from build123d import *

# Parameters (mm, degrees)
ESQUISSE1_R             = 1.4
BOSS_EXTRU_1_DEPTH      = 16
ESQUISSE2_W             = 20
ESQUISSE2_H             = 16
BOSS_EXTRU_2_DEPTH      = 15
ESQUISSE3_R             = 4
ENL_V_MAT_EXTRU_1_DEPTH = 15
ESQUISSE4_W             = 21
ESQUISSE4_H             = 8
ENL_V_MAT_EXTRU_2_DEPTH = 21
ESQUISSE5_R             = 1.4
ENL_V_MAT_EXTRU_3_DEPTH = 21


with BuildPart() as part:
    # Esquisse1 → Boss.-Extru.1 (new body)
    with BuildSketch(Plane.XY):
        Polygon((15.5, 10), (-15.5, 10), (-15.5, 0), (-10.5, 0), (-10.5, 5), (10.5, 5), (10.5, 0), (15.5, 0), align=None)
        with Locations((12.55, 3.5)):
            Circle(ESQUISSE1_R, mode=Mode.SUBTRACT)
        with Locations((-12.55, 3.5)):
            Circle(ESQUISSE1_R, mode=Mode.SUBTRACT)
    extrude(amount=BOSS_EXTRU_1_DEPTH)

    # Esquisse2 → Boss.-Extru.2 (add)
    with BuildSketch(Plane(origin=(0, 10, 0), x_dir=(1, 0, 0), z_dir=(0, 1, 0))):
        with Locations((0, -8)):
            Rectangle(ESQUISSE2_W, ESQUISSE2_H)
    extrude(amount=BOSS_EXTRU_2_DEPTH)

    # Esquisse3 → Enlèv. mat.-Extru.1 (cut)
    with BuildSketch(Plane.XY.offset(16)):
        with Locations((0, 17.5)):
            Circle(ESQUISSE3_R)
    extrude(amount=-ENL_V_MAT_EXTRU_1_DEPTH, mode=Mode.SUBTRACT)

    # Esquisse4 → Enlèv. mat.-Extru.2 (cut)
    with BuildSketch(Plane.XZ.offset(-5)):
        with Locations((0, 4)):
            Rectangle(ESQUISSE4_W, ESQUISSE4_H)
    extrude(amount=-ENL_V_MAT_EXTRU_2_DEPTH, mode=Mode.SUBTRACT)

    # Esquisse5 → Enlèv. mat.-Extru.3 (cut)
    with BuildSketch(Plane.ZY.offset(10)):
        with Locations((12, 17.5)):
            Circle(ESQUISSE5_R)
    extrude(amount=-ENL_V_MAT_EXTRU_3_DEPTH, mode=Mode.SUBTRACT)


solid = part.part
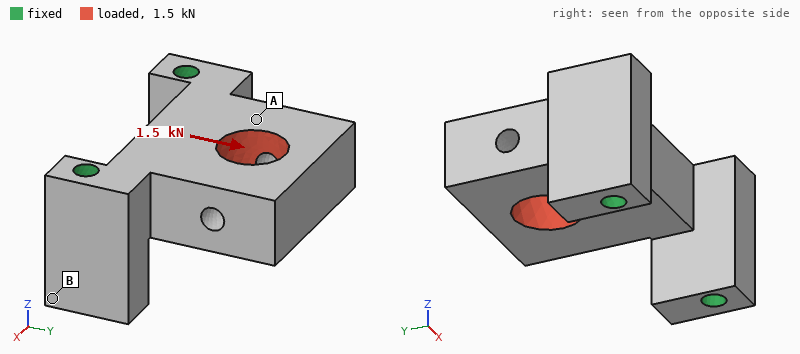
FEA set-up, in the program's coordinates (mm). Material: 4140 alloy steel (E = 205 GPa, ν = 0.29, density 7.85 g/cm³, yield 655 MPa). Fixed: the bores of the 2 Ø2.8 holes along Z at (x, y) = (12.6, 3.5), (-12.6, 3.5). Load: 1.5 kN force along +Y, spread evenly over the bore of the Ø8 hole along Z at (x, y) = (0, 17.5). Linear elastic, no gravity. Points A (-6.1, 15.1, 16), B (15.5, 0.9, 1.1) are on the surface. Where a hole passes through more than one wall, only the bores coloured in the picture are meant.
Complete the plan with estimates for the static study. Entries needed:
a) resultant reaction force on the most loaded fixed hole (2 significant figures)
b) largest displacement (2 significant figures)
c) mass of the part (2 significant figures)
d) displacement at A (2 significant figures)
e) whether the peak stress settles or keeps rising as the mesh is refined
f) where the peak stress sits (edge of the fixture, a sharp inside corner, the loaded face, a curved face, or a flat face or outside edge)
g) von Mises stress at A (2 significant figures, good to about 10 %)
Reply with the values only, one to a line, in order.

880 N
2.8 µm
33 g
1.9 µm
keeps rising
edge of the fixture
17 MPa
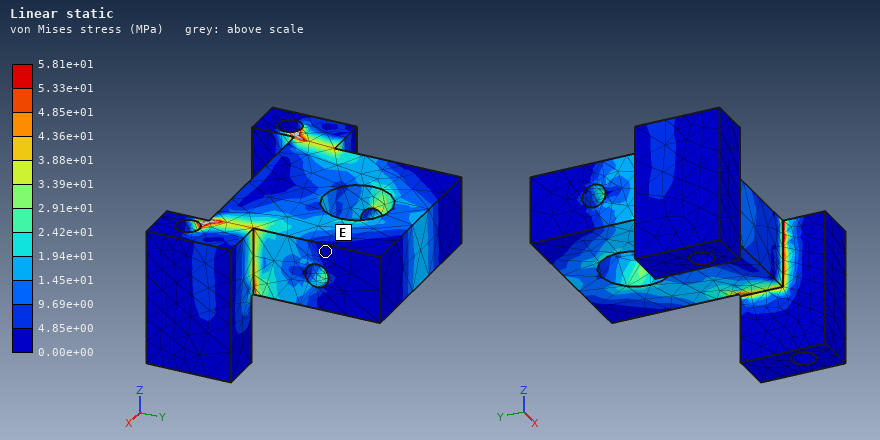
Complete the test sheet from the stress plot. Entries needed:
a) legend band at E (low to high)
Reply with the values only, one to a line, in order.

0.00e+00 to 4.85e+00 MPa
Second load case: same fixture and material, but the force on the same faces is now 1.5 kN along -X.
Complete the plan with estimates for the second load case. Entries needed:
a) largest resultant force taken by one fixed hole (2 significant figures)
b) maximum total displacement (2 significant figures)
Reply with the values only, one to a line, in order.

1.1 kN
5.7 µm
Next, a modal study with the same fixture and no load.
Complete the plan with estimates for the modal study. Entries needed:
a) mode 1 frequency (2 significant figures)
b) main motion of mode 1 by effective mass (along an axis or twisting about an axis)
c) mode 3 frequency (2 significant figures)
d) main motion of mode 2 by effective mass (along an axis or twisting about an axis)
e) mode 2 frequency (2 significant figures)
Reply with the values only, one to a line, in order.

9800 Hz
along Z
25 kHz
along X
24 kHz
